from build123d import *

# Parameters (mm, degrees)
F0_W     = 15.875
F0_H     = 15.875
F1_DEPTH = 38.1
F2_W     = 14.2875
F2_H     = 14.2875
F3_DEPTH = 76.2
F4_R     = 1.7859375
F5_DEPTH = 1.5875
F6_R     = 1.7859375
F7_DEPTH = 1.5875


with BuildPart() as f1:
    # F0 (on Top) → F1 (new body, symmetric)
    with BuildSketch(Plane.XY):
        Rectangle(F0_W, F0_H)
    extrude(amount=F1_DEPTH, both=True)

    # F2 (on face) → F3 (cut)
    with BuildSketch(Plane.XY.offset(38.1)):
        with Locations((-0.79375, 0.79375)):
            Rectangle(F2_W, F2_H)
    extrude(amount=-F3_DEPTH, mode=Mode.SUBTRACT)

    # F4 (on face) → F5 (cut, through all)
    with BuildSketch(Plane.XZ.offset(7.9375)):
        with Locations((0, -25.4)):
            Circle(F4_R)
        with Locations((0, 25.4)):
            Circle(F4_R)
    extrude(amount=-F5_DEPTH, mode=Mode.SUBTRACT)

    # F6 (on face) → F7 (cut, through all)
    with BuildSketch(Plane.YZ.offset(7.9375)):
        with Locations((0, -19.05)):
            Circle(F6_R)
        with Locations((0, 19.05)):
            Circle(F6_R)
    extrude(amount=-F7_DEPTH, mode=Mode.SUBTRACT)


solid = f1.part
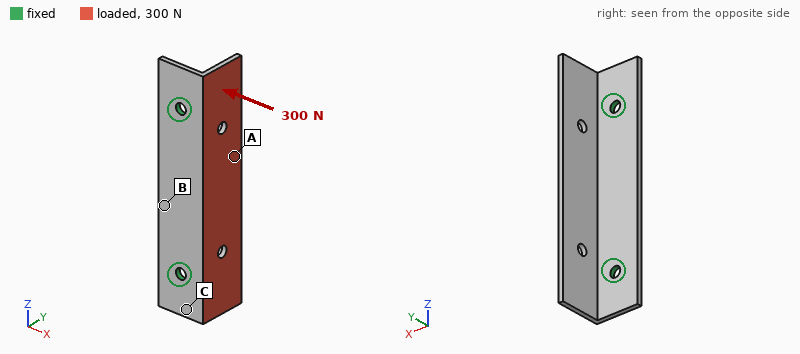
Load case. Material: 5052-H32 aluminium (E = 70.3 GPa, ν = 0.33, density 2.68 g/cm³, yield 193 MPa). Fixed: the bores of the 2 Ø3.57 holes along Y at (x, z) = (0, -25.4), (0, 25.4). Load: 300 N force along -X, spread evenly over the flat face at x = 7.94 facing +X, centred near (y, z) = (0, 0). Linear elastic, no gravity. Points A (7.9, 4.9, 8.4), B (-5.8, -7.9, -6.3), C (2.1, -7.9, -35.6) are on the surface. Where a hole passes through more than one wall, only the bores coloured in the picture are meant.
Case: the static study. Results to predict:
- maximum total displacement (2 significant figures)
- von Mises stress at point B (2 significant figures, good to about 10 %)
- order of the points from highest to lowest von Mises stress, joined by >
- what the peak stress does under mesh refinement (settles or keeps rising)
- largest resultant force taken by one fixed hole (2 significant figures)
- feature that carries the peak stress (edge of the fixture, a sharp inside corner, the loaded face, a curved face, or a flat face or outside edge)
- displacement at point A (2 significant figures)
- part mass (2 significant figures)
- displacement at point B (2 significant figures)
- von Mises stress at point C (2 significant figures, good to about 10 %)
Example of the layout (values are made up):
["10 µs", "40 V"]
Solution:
["0.26 mm", "31 MPa", "C > B > A", "keeps rising", "150 N", "edge of the fixture", "0.21 mm", "9.6 g", "0.085 mm", "49 MPa"]
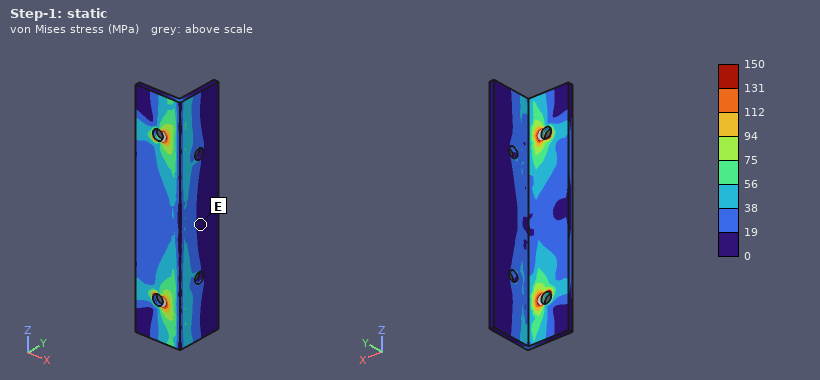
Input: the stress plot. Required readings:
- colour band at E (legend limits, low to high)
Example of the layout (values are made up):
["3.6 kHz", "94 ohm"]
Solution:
["0 to 19 MPa"]
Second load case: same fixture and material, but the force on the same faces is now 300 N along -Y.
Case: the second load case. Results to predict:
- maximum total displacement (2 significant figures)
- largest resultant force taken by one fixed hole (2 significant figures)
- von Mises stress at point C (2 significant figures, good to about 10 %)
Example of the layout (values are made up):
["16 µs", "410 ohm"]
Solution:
["0.13 mm", "150 N", "29 MPa"]
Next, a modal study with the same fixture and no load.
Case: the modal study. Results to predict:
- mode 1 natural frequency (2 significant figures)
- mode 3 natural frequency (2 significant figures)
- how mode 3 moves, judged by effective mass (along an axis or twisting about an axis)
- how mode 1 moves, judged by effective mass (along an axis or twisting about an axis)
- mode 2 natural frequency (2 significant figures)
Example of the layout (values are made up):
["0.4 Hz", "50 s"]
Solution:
["2800 Hz", "5000 Hz", "along Y", "along X", "3900 Hz"]
